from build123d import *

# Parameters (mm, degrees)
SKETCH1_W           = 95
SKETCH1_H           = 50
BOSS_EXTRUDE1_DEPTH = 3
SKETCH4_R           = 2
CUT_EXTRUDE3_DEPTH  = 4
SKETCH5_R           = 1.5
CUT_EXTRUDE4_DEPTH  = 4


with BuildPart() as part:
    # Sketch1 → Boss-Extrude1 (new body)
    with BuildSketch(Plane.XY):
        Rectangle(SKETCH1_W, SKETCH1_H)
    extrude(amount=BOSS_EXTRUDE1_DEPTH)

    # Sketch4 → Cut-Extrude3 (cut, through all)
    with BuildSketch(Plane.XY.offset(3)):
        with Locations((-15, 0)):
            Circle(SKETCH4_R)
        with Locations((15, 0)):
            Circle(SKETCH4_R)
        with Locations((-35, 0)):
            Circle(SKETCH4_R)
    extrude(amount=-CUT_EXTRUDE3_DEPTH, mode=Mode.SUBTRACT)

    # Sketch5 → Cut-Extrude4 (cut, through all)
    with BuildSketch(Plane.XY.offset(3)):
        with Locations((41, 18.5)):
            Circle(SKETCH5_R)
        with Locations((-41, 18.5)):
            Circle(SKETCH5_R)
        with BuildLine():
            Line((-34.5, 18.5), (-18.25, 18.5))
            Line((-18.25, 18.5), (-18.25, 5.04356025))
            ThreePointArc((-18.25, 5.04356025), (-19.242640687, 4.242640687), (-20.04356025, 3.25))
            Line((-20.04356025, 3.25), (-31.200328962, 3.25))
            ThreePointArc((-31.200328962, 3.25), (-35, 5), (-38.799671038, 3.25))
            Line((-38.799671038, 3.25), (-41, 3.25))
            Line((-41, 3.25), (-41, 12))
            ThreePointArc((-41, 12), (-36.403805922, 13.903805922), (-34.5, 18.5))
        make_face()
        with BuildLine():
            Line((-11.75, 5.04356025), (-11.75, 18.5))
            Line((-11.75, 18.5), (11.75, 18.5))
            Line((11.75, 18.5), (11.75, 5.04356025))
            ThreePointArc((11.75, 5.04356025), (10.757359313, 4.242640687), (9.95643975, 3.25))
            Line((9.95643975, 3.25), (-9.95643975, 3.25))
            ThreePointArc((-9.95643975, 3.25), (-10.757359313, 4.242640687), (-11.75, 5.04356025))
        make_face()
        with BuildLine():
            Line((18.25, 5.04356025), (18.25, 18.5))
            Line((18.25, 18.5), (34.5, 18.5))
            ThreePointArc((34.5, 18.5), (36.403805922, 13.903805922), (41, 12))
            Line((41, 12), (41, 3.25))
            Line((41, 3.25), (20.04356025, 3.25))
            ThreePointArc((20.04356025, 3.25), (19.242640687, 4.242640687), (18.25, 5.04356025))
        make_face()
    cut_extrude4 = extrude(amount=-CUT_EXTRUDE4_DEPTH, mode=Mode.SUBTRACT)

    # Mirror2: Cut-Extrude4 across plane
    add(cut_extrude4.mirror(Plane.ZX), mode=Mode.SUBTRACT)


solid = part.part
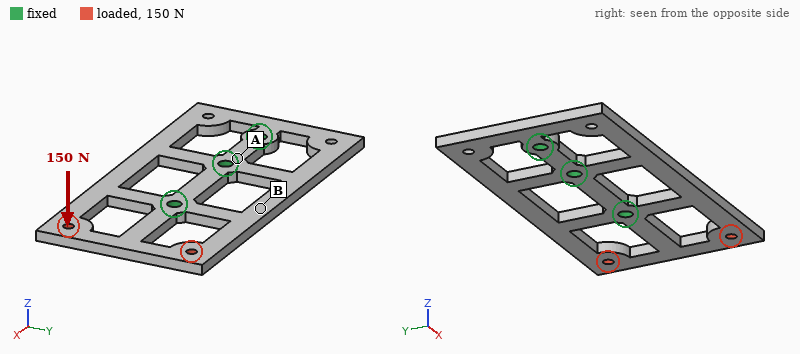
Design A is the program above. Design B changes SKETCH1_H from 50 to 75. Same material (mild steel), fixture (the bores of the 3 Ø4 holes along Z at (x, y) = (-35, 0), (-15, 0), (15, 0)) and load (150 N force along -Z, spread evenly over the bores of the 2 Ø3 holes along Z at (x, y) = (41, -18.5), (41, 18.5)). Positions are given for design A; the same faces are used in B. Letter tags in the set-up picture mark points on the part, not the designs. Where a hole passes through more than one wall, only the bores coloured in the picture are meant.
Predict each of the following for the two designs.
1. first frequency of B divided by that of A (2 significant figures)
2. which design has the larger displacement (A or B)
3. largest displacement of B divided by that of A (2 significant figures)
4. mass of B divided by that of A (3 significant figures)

0.61
A
0.78
1.87
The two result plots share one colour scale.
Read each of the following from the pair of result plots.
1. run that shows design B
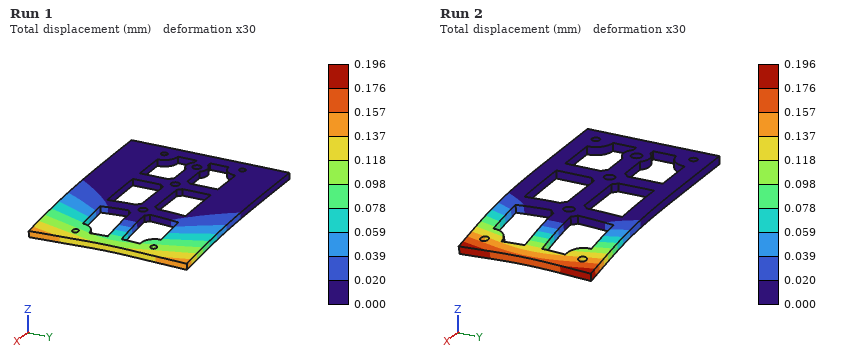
Run 1
